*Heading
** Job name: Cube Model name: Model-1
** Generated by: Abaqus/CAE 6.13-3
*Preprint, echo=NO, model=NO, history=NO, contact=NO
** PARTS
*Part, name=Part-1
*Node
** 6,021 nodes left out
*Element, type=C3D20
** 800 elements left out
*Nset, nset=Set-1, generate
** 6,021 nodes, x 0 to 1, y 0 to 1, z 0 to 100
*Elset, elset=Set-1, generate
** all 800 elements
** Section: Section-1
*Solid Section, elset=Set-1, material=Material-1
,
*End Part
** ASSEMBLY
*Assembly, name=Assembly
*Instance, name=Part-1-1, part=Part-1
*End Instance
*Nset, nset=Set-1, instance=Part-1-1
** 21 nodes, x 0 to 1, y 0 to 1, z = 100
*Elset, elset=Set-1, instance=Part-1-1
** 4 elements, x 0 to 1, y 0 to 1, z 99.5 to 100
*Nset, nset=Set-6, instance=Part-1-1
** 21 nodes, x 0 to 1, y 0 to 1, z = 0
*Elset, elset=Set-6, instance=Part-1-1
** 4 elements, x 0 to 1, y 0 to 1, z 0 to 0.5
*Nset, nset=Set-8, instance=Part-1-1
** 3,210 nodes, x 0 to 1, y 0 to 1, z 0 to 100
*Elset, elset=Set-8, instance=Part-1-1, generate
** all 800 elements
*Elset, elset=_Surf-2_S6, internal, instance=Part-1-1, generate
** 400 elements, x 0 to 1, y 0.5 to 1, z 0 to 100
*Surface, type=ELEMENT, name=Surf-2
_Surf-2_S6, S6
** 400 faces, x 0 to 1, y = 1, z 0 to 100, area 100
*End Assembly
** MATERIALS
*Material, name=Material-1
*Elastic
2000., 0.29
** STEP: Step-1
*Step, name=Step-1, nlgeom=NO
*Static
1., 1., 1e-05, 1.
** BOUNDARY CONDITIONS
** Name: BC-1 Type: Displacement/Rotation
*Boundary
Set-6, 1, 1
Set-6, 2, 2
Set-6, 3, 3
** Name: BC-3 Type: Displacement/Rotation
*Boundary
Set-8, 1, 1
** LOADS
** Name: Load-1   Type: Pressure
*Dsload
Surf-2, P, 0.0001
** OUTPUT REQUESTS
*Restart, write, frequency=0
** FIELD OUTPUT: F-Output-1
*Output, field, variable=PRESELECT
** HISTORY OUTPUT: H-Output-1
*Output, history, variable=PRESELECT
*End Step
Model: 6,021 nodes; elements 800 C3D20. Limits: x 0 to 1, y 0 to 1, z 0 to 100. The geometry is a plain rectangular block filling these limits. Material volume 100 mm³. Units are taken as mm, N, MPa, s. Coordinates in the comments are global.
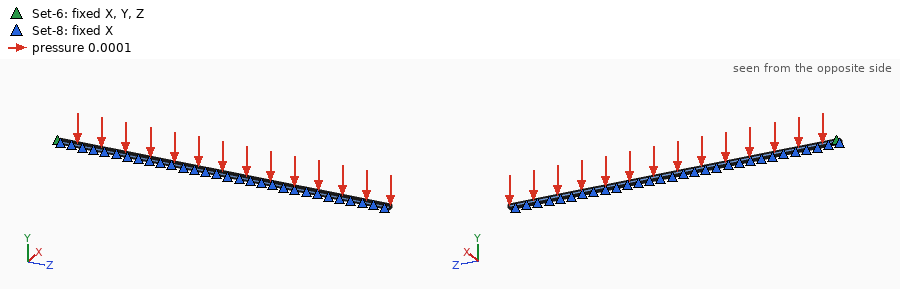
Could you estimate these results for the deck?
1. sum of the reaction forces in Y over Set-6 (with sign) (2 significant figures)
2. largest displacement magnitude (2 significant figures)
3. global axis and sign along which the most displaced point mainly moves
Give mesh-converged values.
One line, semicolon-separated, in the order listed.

0.010 N; 6.9 mm; -Y
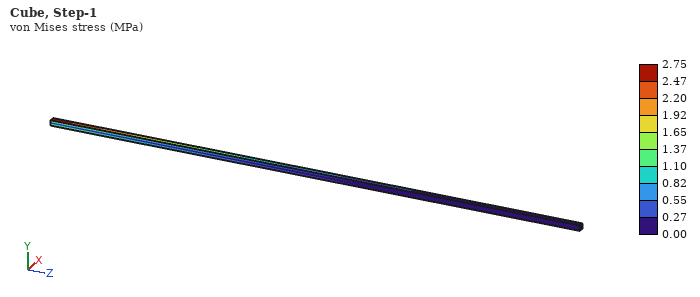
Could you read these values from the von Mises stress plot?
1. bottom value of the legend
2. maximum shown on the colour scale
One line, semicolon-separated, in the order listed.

0.00 MPa; 2.75 MPa
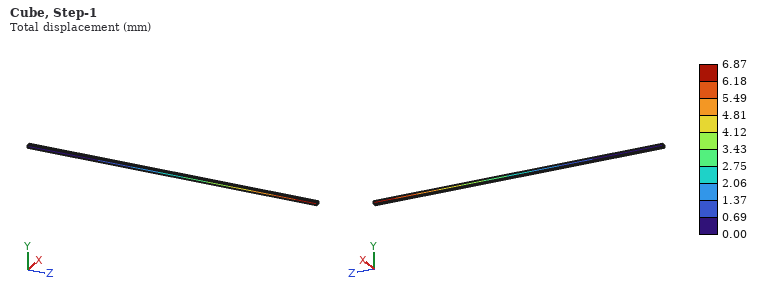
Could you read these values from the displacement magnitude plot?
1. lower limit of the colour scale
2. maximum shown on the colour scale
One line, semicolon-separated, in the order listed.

0.00 mm; 6.87 mm
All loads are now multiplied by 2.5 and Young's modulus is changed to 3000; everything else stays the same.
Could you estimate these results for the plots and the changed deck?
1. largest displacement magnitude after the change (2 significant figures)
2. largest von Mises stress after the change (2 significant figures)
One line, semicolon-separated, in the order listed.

11 mm; 6.9 MPa
